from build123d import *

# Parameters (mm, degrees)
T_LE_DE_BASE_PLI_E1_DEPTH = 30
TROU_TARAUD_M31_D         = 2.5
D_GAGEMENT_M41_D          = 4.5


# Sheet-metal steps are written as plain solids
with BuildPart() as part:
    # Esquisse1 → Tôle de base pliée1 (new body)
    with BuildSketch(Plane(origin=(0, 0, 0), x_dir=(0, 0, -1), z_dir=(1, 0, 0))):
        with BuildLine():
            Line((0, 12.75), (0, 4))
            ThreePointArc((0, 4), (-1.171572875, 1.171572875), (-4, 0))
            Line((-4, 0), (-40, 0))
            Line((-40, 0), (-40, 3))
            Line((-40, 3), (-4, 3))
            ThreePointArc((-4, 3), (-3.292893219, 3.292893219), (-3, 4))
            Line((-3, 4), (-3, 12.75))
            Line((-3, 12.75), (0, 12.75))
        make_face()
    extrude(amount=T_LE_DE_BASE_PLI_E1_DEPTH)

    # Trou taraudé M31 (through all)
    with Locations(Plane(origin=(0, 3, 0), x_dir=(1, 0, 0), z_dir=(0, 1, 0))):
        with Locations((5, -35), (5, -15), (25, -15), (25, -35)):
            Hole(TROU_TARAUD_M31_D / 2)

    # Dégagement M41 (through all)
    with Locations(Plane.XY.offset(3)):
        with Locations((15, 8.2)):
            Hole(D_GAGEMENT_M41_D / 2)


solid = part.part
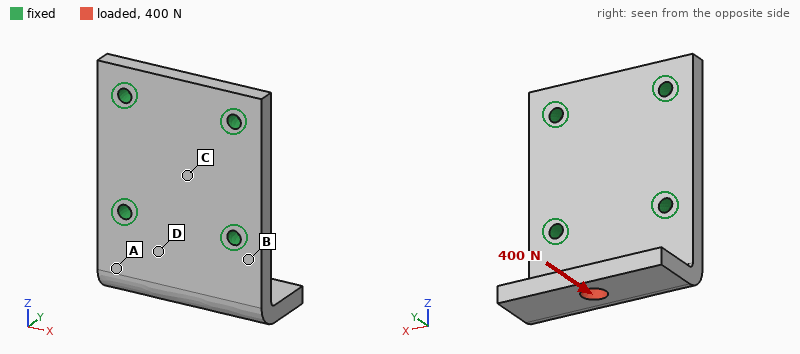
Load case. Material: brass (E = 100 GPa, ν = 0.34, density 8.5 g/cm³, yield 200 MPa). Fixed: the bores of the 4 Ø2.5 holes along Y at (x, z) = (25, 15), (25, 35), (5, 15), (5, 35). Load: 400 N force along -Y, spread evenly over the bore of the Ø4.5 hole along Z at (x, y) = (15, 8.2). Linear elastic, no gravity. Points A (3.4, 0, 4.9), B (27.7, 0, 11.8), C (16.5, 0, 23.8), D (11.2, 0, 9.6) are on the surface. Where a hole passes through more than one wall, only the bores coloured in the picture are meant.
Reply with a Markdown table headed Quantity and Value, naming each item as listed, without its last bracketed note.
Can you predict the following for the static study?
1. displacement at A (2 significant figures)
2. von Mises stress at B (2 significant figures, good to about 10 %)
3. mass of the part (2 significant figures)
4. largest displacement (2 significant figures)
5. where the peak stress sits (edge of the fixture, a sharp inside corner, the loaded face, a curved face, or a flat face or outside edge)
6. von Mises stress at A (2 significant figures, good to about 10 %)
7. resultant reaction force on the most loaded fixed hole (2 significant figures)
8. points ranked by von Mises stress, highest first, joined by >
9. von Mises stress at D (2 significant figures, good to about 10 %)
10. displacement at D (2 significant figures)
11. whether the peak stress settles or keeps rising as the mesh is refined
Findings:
| Quantity | Value |
|---|---|
| displacement at A | 35 µm |
| von Mises stress at B | 94 MPa |
| mass of the part | 36 g |
| largest displacement | 90 µm |
| where the peak stress sits | edge of the fixture |
| von Mises stress at A | 29 MPa |
| resultant reaction force on the most loaded fixed hole | 230 N |
| points ranked by von Mises stress, highest first, joined by > | B > D > A > C |
| von Mises stress at D | 57 MPa |
| displacement at D | 16 µm |
| whether the peak stress settles or keeps rising as the mesh is refined | keeps rising |
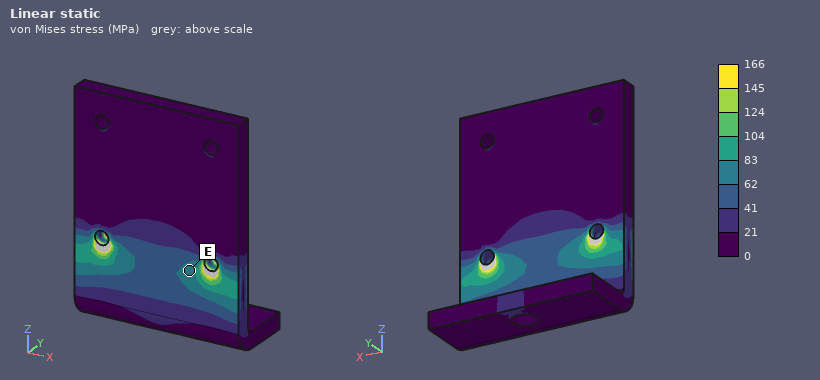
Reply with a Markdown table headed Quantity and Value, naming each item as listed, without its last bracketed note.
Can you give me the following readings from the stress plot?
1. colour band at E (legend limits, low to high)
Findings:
| Quantity | Value |
|---|---|
| colour band at E | 62 to 83 MPa |
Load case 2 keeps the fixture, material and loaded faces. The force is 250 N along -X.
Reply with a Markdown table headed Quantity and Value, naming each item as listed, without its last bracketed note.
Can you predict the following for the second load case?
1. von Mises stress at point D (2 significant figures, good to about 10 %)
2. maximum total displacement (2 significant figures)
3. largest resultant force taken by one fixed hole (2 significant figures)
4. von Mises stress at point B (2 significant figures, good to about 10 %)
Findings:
| Quantity | Value |
|---|---|
| von Mises stress at point D | 7.9 MPa |
| maximum total displacement | 19 µm |
| largest resultant force taken by one fixed hole | 200 N |
| von Mises stress at point B | 24 MPa |
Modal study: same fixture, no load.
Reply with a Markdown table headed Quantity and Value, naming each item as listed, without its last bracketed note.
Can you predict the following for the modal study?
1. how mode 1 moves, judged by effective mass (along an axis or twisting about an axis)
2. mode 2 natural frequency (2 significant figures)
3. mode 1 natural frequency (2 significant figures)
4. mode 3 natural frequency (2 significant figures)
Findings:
| Quantity | Value |
|---|---|
| how mode 1 moves, judged by effective mass | along Y |
| mode 2 natural frequency | 6000 Hz |
| mode 1 natural frequency | 3600 Hz |
| mode 3 natural frequency | 11 kHz |
